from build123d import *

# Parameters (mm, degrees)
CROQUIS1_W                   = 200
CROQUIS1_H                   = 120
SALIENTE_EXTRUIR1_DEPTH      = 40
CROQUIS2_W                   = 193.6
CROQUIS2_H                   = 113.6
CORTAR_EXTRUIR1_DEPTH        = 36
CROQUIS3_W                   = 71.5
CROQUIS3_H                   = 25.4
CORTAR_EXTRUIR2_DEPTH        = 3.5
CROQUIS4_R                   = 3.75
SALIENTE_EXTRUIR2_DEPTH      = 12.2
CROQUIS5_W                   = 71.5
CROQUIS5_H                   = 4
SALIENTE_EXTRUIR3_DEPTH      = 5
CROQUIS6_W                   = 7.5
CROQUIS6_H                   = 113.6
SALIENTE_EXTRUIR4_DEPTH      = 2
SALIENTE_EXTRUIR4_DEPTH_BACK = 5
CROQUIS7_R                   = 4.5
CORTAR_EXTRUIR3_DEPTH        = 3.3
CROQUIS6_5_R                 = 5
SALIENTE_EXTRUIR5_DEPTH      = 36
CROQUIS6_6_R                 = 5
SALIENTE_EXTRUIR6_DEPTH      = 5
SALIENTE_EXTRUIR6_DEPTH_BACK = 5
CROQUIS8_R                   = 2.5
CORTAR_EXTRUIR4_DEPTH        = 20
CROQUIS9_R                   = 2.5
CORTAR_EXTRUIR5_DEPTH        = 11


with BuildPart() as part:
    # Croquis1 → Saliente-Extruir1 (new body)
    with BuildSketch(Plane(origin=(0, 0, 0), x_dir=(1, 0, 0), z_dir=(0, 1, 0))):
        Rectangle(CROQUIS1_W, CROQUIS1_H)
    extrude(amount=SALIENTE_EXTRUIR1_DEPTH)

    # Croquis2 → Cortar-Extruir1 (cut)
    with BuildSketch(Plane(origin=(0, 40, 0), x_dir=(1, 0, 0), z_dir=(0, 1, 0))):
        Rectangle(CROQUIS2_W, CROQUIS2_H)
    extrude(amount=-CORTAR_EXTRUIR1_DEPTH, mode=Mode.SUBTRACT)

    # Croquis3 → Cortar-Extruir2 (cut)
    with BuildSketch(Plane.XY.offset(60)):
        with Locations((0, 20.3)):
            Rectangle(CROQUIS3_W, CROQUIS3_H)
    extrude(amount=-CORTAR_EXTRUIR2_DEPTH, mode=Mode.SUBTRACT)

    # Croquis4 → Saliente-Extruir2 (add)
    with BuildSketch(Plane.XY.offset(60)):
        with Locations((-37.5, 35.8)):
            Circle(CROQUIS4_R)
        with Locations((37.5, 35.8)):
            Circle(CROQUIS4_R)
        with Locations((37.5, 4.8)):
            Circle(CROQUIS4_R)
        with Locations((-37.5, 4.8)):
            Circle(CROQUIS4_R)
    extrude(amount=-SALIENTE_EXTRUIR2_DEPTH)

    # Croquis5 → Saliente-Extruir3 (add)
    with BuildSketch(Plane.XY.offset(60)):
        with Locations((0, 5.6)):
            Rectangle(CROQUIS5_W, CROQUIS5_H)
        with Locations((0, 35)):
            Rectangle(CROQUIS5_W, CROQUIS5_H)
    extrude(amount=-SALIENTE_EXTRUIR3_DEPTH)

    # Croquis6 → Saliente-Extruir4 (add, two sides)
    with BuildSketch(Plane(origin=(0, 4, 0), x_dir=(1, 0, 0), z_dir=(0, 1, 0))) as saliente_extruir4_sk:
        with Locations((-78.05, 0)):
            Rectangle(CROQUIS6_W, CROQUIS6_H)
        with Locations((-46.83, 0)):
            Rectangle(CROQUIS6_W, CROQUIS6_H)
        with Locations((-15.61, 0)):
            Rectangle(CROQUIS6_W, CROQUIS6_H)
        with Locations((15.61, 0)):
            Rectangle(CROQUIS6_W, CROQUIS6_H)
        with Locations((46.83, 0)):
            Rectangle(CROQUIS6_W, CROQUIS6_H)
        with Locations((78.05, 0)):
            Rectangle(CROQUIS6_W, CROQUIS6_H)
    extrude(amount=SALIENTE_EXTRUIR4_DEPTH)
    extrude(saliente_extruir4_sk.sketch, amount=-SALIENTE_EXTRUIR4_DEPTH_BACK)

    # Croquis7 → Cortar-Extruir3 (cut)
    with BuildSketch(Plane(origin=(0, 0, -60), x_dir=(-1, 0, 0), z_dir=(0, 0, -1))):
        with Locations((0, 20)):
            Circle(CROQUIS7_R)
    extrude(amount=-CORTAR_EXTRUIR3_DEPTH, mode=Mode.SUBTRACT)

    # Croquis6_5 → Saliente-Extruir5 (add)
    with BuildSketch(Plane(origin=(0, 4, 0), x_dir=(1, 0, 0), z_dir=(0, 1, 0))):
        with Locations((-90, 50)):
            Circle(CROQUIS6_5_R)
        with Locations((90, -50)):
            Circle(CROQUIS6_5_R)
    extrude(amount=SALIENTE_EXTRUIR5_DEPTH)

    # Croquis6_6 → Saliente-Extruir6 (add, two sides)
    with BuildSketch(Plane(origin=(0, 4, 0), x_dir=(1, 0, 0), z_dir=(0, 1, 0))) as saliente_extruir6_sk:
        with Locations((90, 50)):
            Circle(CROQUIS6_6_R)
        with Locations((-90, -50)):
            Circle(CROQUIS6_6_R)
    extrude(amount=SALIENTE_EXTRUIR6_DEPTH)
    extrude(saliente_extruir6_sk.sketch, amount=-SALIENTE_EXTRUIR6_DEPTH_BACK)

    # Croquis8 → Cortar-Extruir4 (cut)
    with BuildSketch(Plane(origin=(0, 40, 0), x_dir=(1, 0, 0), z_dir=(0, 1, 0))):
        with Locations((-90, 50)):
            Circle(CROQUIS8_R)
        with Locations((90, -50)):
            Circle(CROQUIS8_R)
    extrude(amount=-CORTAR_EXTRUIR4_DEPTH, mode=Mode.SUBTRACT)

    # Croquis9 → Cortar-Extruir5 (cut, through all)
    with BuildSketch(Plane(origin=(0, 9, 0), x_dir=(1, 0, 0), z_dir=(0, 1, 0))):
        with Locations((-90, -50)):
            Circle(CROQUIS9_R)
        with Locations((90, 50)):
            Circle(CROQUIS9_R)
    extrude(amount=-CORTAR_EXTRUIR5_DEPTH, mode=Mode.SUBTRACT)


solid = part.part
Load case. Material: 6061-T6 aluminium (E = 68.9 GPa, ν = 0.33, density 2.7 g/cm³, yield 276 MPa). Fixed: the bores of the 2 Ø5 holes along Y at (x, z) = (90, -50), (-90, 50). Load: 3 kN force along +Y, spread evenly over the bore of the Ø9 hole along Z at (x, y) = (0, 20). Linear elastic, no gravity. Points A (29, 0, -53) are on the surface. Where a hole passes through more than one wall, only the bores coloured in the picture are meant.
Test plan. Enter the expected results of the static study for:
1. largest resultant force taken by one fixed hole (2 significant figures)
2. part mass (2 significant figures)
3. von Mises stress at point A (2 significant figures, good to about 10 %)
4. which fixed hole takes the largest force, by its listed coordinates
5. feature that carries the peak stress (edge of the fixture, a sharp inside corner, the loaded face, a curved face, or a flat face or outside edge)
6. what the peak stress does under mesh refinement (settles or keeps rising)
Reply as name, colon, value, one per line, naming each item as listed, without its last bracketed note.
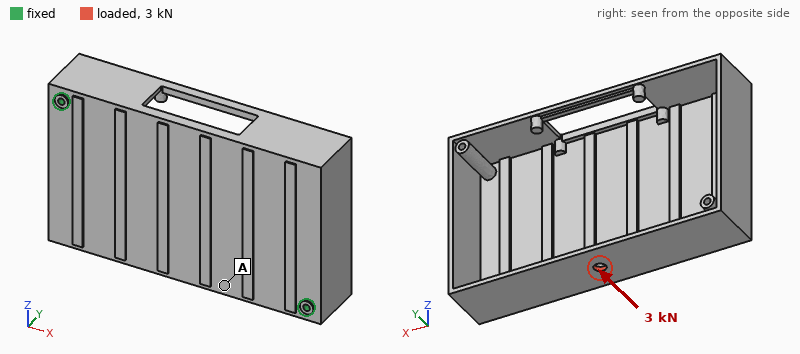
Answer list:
largest resultant force taken by one fixed hole: 2.0 kN
part mass: 500 g
von Mises stress at point A: 37 MPa
which fixed hole takes the largest force, by its listed coordinates: (90, -50)
feature that carries the peak stress: edge of the fixture
what the peak stress does under mesh refinement: keeps rising
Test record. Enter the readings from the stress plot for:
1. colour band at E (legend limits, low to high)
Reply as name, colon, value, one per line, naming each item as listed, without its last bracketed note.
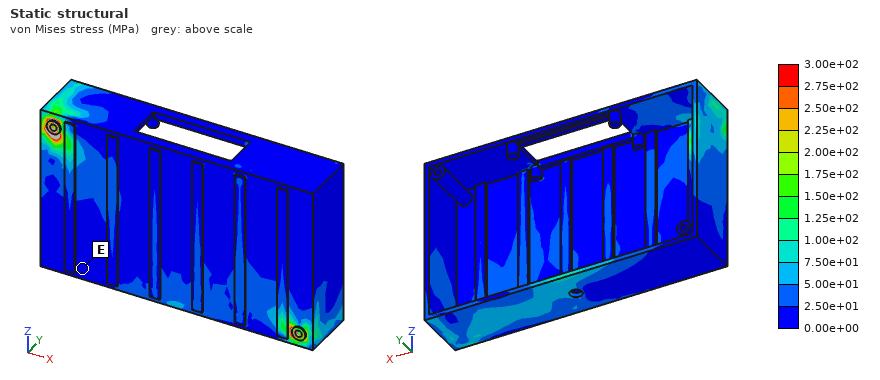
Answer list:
colour band at E: 0.00e+00 to 2.50e+01 MPa
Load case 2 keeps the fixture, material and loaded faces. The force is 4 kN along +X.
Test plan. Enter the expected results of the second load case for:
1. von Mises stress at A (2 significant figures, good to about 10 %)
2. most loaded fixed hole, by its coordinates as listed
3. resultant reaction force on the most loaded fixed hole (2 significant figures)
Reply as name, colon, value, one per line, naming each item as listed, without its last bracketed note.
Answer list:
von Mises stress at A: 13 MPa
most loaded fixed hole, by its coordinates as listed: (90, -50)
resultant reaction force on the most loaded fixed hole: 3.1 kN
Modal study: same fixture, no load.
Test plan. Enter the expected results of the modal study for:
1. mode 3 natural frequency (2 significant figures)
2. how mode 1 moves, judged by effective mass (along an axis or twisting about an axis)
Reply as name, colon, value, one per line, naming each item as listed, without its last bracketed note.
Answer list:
mode 3 natural frequency: 1200 Hz
how mode 1 moves, judged by effective mass: along Y
